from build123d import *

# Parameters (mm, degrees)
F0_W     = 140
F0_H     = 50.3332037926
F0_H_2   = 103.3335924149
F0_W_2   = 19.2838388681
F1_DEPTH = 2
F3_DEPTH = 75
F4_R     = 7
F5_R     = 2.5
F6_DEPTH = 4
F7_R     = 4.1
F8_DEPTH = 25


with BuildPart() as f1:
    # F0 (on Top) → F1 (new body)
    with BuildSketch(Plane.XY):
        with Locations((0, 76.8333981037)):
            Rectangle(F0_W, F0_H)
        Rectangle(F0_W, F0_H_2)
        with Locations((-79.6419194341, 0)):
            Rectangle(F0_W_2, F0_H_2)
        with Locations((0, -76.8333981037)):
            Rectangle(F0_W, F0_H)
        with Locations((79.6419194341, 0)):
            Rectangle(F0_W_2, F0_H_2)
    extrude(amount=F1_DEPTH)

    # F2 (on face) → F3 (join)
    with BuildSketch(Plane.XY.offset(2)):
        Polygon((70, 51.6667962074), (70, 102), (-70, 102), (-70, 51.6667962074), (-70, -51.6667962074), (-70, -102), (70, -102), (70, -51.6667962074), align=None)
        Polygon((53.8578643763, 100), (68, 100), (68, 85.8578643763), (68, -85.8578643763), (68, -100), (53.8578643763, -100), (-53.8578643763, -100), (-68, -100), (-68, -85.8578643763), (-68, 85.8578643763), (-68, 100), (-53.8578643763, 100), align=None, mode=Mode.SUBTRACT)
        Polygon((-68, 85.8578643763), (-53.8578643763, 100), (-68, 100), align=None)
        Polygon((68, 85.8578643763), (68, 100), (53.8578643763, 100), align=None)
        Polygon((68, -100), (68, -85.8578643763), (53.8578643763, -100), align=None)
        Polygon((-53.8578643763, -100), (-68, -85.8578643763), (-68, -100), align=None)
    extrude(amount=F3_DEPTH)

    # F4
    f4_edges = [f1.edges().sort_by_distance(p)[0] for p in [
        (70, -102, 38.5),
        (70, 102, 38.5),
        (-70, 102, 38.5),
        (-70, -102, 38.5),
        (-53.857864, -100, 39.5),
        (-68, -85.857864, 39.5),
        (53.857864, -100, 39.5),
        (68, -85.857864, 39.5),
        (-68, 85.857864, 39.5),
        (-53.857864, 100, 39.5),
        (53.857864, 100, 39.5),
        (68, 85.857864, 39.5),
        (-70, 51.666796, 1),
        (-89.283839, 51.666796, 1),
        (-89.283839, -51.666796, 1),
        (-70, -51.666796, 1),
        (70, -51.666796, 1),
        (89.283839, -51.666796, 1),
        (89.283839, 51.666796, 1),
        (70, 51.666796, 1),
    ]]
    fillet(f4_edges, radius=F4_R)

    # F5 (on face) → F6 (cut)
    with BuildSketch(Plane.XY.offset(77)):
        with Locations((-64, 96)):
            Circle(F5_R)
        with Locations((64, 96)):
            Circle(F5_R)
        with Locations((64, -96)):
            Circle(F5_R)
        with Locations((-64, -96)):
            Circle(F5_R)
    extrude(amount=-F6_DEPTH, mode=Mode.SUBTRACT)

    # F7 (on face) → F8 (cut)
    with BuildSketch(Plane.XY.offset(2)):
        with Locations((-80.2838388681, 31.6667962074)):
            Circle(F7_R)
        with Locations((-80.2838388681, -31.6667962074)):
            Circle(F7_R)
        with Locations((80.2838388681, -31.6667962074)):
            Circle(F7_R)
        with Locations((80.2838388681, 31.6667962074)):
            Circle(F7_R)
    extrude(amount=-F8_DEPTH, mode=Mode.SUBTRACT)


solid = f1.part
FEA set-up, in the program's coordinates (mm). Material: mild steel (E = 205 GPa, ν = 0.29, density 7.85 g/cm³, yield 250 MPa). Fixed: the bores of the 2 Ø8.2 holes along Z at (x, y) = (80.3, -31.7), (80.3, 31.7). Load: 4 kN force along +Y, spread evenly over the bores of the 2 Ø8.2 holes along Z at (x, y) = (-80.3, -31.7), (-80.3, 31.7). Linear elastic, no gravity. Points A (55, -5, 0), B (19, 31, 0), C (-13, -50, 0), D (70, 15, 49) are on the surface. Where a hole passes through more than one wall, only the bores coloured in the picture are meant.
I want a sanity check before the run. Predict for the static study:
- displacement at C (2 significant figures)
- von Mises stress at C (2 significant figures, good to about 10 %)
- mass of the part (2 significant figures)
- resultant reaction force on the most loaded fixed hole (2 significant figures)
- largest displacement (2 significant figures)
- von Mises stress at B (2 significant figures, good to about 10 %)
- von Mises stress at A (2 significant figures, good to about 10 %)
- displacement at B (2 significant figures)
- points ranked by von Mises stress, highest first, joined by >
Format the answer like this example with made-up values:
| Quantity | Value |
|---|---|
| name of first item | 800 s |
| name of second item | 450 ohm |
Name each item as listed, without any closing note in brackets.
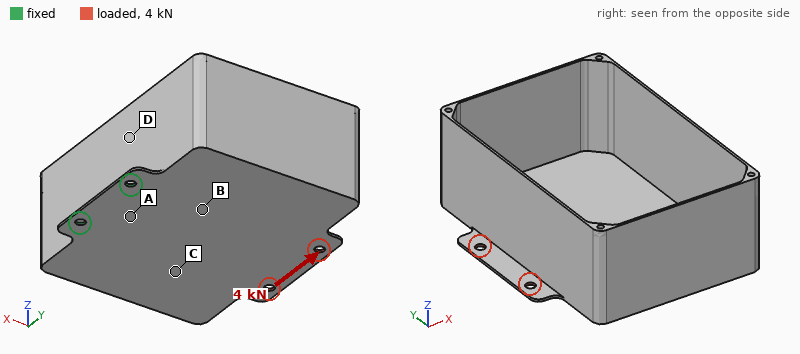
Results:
| Quantity | Value |
|---|---|
| displacement at C | 0.12 mm |
| von Mises stress at C | 26 MPa |
| mass of the part | 1.5 kg |
| resultant reaction force on the most loaded fixed hole | 9.5 kN |
| largest displacement | 0.21 mm |
| von Mises stress at B | 52 MPa |
| von Mises stress at A | 91 MPa |
| displacement at B | 0.072 mm |
| points ranked by von Mises stress, highest first, joined by > | A > B > C > D |
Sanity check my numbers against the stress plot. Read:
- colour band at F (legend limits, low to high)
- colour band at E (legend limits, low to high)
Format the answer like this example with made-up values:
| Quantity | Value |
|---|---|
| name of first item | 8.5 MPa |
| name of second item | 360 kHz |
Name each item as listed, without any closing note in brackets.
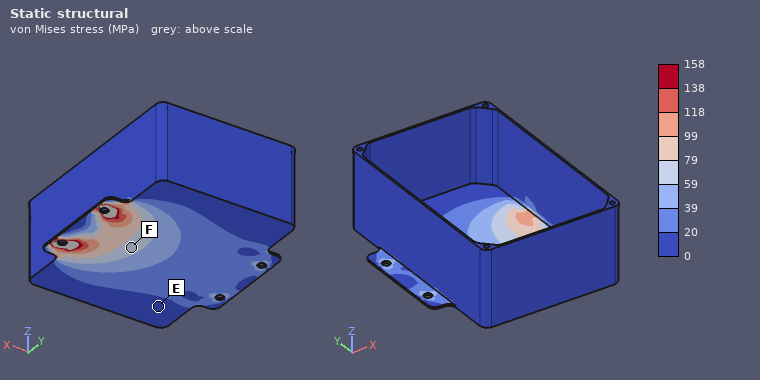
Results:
| Quantity | Value |
|---|---|
| colour band at F | 59 to 79 MPa |
| colour band at E | 0 to 20 MPa |
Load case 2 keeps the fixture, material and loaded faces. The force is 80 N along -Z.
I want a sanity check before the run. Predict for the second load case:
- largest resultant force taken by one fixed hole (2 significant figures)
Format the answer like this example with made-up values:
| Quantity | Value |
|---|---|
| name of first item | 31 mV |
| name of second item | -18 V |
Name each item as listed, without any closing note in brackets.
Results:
| Quantity | Value |
|---|---|
| largest resultant force taken by one fixed hole | 44 N |
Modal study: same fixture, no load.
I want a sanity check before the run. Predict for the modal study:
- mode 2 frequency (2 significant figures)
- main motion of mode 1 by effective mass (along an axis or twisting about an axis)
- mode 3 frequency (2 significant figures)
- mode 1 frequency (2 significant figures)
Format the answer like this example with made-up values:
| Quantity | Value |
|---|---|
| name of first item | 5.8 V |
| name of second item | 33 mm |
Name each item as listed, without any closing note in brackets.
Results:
| Quantity | Value |
|---|---|
| mode 2 frequency | 94 Hz |
| main motion of mode 1 by effective mass | along Z |
| mode 3 frequency | 440 Hz |
| mode 1 frequency | 36 Hz |
